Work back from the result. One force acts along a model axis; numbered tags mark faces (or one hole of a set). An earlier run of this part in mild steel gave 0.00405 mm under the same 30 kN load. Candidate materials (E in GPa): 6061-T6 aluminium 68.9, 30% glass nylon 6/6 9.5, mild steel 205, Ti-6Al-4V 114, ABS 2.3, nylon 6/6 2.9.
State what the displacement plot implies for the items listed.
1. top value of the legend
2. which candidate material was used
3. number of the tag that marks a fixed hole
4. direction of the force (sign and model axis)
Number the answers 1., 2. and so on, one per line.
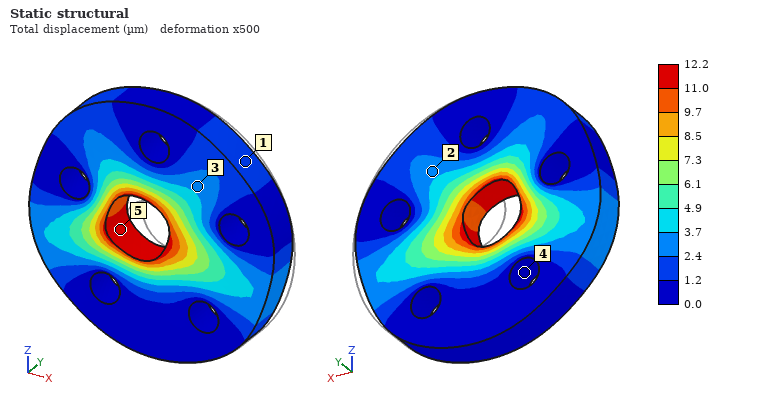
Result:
1. 12.2 µm
2. 6061-T6 aluminium
3. 4
4. -X
